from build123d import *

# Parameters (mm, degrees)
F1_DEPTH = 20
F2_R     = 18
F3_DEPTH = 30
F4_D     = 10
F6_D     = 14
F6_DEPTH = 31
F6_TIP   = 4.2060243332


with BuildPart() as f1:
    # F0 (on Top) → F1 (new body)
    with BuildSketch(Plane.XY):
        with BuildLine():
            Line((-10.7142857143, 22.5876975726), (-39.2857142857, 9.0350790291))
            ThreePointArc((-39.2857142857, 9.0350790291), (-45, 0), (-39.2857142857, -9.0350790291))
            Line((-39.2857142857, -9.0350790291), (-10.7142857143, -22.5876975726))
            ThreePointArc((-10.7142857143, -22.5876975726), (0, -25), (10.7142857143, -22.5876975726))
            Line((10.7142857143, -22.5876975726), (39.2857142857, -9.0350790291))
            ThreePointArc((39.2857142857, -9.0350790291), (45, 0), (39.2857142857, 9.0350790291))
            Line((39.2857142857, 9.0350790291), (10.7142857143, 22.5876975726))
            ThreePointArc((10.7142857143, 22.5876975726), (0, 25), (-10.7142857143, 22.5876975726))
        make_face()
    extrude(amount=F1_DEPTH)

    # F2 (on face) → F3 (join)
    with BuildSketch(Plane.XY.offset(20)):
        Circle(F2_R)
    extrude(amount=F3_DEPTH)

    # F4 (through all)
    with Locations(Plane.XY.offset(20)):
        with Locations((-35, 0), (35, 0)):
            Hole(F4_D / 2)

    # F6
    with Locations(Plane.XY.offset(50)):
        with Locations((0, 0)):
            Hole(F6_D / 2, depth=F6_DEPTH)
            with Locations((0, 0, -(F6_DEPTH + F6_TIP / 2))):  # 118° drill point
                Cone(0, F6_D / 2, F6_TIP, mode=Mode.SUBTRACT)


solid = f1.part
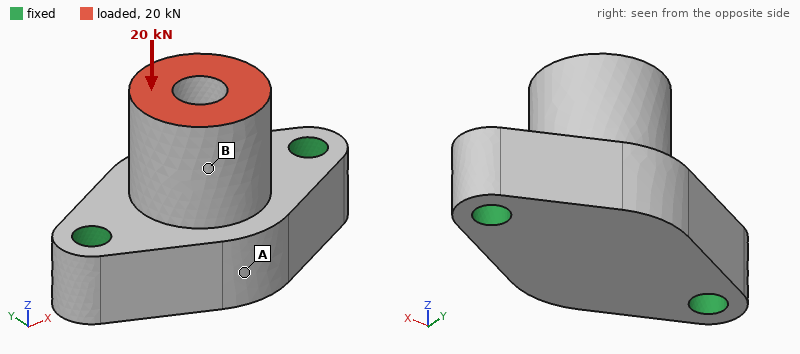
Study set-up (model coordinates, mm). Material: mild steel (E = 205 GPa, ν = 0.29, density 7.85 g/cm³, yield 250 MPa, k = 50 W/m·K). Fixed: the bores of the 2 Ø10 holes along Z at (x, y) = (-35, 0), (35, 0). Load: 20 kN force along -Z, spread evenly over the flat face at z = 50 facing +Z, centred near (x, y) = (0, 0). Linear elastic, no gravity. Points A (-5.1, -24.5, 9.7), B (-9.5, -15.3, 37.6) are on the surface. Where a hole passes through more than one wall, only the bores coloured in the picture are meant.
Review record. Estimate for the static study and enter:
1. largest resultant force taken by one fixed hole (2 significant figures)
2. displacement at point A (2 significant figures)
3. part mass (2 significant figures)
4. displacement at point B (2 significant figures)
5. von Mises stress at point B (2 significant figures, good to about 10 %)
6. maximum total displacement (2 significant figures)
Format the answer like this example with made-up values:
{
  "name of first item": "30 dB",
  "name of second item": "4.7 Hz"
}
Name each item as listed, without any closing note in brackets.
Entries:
{
  "largest resultant force taken by one fixed hole": "10 kN",
  "displacement at point A": "9.2 µm",
  "part mass": "650 g",
  "displacement at point B": "10 µm",
  "von Mises stress at point B": "21 MPa",
  "maximum total displacement": "12 µm"
}
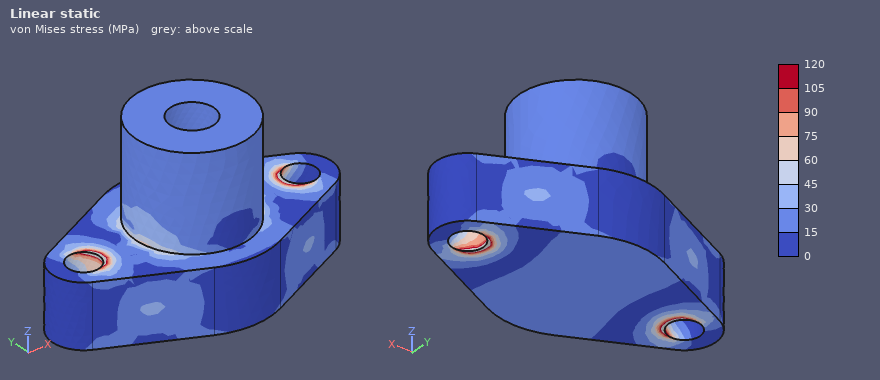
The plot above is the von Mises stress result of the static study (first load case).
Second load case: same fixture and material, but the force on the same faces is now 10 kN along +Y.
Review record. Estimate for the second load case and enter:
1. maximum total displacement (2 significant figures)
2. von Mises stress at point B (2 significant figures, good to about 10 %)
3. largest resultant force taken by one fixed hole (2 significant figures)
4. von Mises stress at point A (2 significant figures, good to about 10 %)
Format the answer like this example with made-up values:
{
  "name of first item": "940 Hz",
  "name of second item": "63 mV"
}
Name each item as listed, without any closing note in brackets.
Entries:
{
  "maximum total displacement": "64 µm",
  "von Mises stress at point B": "30 MPa",
  "largest resultant force taken by one fixed hole": "5.0 kN",
  "von Mises stress at point A": "18 MPa"
}
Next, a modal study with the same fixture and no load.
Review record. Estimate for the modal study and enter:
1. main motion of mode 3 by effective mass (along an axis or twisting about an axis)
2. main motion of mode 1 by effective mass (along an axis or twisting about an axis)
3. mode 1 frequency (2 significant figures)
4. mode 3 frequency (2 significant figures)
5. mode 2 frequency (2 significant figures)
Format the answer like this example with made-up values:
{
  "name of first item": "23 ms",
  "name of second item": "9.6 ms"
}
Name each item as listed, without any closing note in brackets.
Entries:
{
  "main motion of mode 3 by effective mass": "along X",
  "main motion of mode 1 by effective mass": "along Y",
  "mode 1 frequency": "6100 Hz",
  "mode 3 frequency": "11 kHz",
  "mode 2 frequency": "11 kHz"
}
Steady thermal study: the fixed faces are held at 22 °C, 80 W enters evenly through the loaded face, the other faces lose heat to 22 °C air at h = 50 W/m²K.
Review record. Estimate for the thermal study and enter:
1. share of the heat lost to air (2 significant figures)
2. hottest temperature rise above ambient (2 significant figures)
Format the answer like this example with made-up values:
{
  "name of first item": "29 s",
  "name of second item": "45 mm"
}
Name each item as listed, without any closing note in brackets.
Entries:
{
  "share of the heat lost to air": "23 %",
  "hottest temperature rise above ambient": "79 K"
}
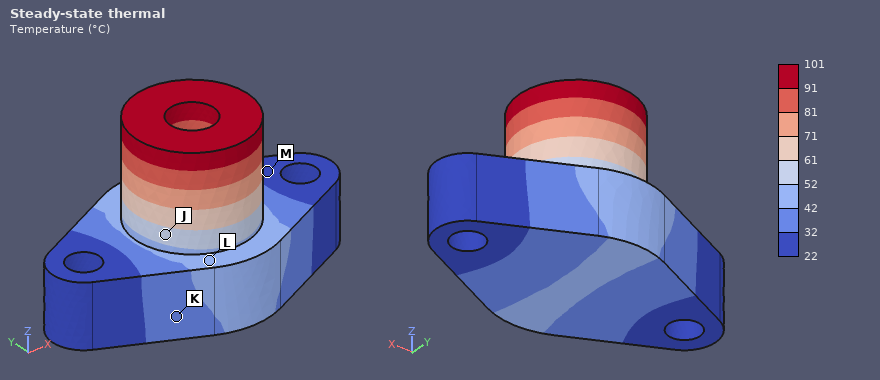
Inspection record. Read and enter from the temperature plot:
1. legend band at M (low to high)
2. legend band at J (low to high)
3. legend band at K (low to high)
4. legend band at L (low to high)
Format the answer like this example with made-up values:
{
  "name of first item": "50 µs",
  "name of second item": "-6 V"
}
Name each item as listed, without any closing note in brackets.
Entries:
{
  "legend band at M": "22 to 32 °C",
  "legend band at J": "52 to 61 °C",
  "legend band at K": "32 to 42 °C",
  "legend band at L": "42 to 52 °C"
}
